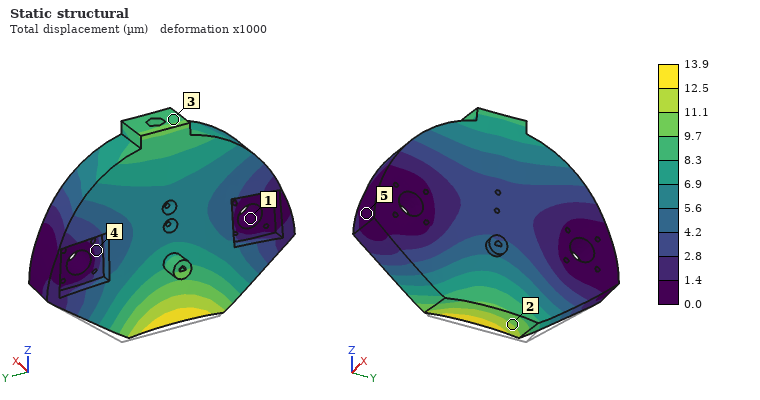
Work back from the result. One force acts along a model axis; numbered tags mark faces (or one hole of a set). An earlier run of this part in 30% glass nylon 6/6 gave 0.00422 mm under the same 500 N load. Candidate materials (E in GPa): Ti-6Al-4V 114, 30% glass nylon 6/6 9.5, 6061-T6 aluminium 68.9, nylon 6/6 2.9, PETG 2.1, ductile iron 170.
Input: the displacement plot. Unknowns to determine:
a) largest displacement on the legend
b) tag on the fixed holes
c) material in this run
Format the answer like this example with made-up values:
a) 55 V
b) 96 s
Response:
a) 13.9 µm
b) 1
c) nylon 6/6
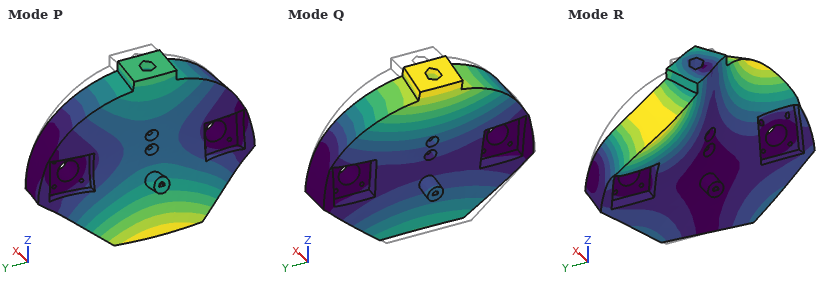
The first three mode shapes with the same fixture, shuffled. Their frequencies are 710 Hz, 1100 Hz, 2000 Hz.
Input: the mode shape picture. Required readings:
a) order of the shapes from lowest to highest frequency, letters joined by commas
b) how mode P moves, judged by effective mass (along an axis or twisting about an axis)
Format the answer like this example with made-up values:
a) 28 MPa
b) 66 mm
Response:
a) Q, P, R
b) along X
